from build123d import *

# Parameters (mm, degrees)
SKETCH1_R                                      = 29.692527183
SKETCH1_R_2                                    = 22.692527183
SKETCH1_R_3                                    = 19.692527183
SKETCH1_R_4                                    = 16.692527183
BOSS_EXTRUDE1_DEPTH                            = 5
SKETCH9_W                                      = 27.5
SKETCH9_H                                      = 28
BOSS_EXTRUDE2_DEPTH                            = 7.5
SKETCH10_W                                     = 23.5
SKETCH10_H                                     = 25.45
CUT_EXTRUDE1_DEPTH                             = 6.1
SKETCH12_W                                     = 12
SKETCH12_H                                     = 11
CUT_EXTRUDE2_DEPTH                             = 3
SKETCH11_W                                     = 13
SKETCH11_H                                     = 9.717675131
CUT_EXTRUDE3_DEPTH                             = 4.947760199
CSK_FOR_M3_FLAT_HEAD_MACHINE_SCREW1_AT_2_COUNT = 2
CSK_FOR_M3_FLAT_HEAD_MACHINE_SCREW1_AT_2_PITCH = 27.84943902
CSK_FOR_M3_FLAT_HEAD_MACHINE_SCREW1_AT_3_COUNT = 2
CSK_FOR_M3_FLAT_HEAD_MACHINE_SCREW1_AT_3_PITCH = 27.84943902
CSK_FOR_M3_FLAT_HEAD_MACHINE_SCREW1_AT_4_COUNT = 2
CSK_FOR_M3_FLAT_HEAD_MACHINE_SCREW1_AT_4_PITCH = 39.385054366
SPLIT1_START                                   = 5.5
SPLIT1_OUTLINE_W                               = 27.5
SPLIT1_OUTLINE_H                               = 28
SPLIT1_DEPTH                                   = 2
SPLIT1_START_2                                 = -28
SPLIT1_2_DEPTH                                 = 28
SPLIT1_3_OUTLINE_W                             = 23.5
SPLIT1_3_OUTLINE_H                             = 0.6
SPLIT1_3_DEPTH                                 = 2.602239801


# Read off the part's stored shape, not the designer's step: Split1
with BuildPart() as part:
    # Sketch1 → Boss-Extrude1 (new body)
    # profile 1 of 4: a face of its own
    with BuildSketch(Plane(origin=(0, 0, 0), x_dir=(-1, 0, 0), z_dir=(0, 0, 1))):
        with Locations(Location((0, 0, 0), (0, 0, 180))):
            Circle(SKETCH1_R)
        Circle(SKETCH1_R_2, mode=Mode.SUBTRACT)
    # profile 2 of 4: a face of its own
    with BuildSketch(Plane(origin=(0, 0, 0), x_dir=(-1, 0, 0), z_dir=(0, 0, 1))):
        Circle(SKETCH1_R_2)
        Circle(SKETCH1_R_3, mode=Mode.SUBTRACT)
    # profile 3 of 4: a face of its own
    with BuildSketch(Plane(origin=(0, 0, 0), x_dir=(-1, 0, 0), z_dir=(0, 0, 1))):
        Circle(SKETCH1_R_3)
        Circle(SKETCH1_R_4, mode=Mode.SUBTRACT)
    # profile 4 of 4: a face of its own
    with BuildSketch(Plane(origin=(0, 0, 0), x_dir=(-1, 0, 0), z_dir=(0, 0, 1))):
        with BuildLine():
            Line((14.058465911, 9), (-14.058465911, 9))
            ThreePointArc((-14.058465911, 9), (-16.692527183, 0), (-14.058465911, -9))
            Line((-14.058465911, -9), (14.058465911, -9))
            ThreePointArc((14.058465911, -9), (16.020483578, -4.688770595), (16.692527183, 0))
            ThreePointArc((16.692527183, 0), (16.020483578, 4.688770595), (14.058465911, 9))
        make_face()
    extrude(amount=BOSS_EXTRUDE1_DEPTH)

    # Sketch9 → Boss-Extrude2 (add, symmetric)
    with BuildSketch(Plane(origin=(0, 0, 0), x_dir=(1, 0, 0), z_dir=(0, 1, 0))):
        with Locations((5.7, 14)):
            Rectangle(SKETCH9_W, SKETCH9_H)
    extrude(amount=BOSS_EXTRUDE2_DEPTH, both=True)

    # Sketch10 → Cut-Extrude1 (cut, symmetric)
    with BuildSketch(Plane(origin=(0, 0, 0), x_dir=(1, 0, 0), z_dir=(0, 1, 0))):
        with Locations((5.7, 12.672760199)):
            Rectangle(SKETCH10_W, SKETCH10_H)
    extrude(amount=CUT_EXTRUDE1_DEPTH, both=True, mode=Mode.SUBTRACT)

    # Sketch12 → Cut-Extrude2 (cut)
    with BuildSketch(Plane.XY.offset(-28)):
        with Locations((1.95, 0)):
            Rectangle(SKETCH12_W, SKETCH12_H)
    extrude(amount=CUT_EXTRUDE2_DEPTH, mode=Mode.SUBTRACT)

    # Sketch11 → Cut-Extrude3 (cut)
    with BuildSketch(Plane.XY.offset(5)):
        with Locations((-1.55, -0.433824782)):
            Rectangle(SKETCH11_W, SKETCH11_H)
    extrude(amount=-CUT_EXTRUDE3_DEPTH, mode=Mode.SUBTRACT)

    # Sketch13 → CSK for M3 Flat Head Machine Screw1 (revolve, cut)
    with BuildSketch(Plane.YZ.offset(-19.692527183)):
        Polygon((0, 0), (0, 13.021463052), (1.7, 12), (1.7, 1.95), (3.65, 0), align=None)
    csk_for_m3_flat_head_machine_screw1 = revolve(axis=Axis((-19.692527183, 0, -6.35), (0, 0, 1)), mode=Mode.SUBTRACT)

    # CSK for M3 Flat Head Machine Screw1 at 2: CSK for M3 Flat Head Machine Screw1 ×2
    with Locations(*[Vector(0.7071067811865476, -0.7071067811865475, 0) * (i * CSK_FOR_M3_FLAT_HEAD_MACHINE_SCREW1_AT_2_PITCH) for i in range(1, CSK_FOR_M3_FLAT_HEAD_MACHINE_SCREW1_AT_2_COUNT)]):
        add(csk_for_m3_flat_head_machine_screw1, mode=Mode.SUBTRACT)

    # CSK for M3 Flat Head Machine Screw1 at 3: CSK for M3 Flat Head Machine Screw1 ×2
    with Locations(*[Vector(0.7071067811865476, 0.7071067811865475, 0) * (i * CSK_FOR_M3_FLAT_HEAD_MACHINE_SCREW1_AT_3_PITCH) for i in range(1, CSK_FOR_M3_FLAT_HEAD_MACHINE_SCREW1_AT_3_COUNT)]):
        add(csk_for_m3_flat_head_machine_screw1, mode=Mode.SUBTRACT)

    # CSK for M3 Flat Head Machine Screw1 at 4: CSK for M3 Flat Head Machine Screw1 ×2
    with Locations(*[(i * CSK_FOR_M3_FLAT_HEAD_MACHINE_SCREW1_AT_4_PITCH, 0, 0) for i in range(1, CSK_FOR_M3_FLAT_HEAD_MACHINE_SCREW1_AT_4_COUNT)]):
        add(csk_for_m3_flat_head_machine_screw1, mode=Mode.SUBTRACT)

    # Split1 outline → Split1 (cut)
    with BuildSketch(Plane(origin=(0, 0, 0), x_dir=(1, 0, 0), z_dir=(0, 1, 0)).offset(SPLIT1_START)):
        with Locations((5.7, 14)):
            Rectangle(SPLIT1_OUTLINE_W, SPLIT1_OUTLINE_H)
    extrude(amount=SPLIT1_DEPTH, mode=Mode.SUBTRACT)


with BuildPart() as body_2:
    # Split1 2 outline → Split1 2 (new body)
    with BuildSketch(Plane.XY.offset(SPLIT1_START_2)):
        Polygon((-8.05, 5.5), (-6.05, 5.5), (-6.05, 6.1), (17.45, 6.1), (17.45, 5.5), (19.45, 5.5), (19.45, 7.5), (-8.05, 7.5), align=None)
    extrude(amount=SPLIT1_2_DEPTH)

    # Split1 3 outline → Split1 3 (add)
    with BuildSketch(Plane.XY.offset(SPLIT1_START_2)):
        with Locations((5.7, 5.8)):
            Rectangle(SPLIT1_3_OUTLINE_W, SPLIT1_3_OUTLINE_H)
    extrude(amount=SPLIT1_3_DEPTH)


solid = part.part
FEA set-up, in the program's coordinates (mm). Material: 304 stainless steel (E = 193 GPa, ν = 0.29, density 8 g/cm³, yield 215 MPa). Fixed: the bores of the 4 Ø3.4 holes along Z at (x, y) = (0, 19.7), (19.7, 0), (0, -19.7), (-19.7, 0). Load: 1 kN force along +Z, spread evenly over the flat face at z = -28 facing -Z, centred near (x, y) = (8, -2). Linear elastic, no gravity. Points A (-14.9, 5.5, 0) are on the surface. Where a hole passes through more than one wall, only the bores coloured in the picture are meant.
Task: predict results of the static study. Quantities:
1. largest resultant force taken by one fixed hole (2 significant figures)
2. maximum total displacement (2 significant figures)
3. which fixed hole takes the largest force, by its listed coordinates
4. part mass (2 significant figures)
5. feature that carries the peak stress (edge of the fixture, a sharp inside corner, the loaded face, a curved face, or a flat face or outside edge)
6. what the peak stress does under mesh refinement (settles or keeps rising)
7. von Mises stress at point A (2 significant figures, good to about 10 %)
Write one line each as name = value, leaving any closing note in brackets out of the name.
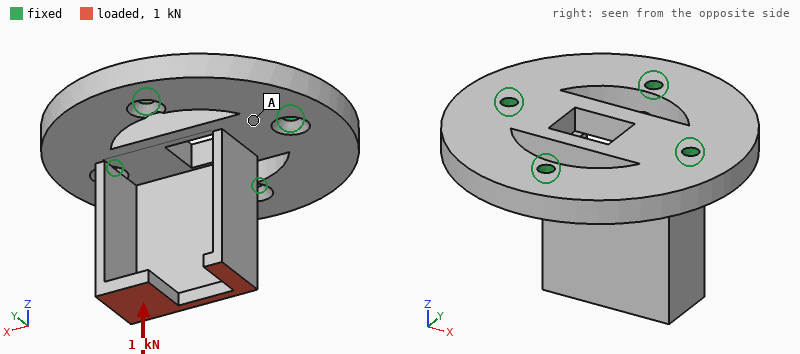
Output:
largest resultant force taken by one fixed hole = 640 N
maximum total displacement = 37 µm
which fixed hole takes the largest force, by its listed coordinates = (19.7, 0)
part mass = 110 g
feature that carries the peak stress = a sharp inside corner
what the peak stress does under mesh refinement = keeps rising
von Mises stress at point A = 13 MPa
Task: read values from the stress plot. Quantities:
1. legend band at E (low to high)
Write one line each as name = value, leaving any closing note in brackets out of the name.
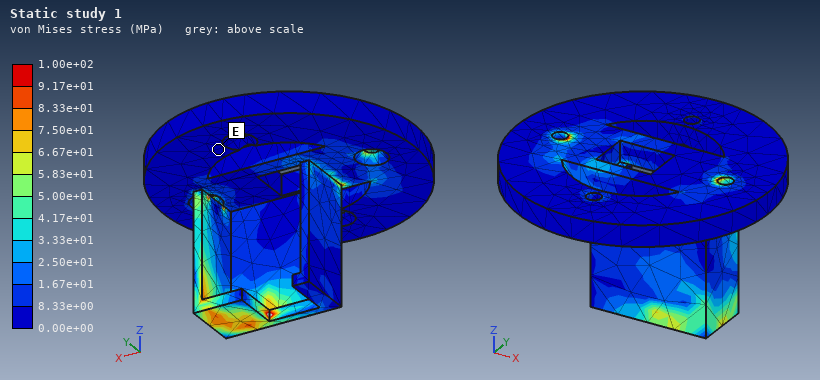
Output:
legend band at E = 0.00e+00 to 8.33e+00 MPa
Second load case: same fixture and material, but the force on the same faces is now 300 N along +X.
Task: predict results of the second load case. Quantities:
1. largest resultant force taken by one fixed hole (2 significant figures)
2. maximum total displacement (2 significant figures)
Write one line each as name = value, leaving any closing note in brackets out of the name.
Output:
largest resultant force taken by one fixed hole = 290 N
maximum total displacement = 48 µm
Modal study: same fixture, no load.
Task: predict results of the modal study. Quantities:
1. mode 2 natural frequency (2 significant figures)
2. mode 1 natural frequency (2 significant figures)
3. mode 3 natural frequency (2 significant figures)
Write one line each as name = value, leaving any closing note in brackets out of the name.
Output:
mode 2 natural frequency = 4900 Hz
mode 1 natural frequency = 4200 Hz
mode 3 natural frequency = 6300 Hz
